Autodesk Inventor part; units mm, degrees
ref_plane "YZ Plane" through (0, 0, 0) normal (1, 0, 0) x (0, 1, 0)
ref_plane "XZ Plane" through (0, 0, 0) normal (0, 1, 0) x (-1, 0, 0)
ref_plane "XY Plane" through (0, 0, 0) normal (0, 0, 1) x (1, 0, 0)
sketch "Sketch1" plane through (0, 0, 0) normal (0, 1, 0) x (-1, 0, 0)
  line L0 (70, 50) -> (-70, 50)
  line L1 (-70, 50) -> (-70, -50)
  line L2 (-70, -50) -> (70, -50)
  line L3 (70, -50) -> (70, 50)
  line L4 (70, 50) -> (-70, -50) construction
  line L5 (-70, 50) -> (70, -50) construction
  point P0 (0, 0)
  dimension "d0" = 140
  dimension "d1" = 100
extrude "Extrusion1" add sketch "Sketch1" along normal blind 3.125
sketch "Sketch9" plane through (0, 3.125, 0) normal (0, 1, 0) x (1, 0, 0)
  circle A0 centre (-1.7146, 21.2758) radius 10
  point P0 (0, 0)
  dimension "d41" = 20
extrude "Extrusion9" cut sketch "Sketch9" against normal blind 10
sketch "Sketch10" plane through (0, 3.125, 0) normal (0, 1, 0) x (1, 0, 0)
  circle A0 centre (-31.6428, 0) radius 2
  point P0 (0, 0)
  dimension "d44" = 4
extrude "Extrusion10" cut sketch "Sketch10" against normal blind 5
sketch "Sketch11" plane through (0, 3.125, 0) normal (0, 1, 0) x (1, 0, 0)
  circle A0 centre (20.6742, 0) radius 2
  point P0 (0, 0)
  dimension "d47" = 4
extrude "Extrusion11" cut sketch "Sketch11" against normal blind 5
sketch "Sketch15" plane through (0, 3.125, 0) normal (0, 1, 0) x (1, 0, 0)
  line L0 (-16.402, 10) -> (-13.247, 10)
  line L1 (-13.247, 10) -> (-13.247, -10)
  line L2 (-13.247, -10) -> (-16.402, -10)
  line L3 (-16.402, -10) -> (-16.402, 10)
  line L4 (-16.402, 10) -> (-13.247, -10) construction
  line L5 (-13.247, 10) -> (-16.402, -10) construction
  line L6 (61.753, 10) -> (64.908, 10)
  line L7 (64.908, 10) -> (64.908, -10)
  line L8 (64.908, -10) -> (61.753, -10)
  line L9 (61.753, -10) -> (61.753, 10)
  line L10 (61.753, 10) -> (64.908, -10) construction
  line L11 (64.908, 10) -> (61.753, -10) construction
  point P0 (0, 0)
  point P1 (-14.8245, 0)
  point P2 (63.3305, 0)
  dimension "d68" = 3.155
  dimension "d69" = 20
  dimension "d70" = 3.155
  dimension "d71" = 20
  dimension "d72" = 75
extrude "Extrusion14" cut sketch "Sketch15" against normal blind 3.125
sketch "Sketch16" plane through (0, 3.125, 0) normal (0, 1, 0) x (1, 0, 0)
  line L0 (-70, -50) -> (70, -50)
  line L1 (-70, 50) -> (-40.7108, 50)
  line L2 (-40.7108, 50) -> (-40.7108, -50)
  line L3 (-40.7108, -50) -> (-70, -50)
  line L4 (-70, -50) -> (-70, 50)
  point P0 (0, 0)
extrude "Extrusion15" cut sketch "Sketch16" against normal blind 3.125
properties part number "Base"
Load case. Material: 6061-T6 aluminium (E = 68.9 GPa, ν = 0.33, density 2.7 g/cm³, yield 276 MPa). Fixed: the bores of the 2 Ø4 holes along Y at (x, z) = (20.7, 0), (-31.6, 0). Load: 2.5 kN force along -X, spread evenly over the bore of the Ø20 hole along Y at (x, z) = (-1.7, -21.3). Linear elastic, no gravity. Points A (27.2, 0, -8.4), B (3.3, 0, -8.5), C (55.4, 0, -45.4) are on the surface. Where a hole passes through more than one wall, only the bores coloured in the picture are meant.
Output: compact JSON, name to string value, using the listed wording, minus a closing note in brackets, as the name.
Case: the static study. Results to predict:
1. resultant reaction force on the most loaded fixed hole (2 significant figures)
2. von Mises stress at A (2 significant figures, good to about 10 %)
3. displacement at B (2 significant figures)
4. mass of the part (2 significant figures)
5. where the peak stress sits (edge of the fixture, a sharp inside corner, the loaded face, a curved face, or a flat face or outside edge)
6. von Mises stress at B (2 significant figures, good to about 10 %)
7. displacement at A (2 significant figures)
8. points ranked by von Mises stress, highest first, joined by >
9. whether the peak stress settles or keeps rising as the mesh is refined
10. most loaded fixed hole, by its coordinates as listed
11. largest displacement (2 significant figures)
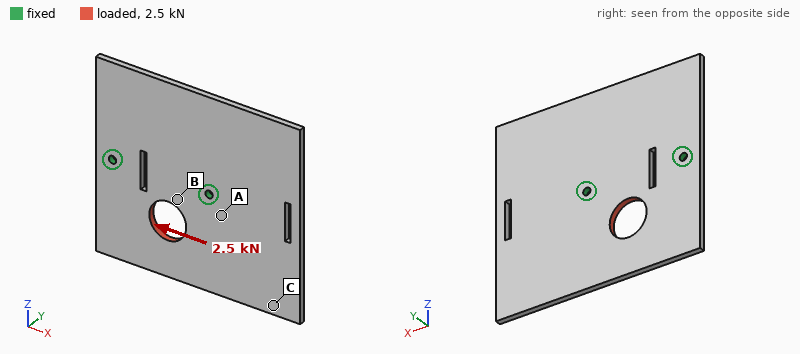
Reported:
{"resultant reaction force on the most loaded fixed hole": "1.9 kN", "von Mises stress at A": "11 MPa", "displacement at B": "8.4 µm", "mass of the part": "89 g", "where the peak stress sits": "edge of the fixture", "von Mises stress at B": "27 MPa", "displacement at A": "8.1 µm", "points ranked by von Mises stress, highest first, joined by >": "B > A > C", "whether the peak stress settles or keeps rising as the mesh is refined": "keeps rising", "most loaded fixed hole, by its coordinates as listed": "(20.7, 0)", "largest displacement": "30 µm"}
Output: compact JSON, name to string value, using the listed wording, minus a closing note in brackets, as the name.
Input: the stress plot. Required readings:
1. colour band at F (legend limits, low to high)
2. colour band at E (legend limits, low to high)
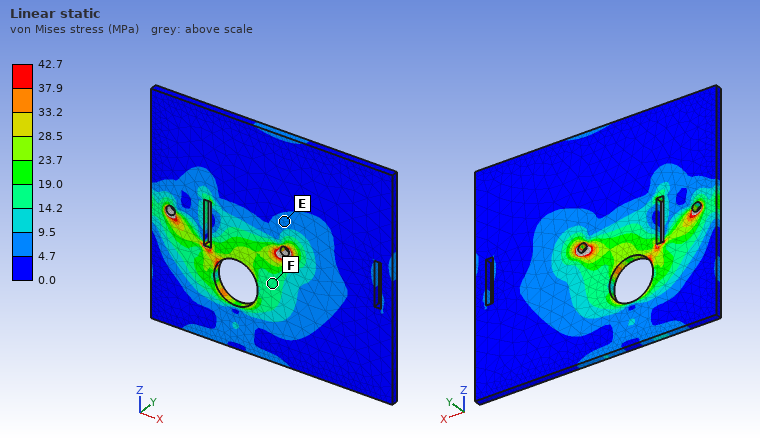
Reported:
{"colour band at F": "14.2 to 19.0 MPa", "colour band at E": "4.7 to 9.5 MPa"}
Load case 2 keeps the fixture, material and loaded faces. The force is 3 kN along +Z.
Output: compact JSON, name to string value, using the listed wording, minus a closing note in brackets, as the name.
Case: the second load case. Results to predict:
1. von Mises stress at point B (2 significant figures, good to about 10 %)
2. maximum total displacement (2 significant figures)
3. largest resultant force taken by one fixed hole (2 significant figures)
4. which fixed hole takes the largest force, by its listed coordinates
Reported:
{"von Mises stress at point B": "14 MPa", "maximum total displacement": "15 µm", "largest resultant force taken by one fixed hole": "1.7 kN", "which fixed hole takes the largest force, by its listed coordinates": "(20.7, 0)"}
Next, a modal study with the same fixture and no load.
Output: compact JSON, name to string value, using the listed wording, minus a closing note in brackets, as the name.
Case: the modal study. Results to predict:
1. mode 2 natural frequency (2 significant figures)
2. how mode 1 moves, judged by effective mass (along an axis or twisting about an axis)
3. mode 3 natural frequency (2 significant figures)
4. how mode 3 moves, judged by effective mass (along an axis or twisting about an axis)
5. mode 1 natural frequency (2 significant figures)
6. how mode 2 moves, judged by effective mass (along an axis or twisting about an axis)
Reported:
{"mode 2 natural frequency": "770 Hz", "how mode 1 moves, judged by effective mass": "twisting about X", "mode 3 natural frequency": "1100 Hz", "how mode 3 moves, judged by effective mass": "along Y", "mode 1 natural frequency": "650 Hz", "how mode 2 moves, judged by effective mass": "along Y"}
